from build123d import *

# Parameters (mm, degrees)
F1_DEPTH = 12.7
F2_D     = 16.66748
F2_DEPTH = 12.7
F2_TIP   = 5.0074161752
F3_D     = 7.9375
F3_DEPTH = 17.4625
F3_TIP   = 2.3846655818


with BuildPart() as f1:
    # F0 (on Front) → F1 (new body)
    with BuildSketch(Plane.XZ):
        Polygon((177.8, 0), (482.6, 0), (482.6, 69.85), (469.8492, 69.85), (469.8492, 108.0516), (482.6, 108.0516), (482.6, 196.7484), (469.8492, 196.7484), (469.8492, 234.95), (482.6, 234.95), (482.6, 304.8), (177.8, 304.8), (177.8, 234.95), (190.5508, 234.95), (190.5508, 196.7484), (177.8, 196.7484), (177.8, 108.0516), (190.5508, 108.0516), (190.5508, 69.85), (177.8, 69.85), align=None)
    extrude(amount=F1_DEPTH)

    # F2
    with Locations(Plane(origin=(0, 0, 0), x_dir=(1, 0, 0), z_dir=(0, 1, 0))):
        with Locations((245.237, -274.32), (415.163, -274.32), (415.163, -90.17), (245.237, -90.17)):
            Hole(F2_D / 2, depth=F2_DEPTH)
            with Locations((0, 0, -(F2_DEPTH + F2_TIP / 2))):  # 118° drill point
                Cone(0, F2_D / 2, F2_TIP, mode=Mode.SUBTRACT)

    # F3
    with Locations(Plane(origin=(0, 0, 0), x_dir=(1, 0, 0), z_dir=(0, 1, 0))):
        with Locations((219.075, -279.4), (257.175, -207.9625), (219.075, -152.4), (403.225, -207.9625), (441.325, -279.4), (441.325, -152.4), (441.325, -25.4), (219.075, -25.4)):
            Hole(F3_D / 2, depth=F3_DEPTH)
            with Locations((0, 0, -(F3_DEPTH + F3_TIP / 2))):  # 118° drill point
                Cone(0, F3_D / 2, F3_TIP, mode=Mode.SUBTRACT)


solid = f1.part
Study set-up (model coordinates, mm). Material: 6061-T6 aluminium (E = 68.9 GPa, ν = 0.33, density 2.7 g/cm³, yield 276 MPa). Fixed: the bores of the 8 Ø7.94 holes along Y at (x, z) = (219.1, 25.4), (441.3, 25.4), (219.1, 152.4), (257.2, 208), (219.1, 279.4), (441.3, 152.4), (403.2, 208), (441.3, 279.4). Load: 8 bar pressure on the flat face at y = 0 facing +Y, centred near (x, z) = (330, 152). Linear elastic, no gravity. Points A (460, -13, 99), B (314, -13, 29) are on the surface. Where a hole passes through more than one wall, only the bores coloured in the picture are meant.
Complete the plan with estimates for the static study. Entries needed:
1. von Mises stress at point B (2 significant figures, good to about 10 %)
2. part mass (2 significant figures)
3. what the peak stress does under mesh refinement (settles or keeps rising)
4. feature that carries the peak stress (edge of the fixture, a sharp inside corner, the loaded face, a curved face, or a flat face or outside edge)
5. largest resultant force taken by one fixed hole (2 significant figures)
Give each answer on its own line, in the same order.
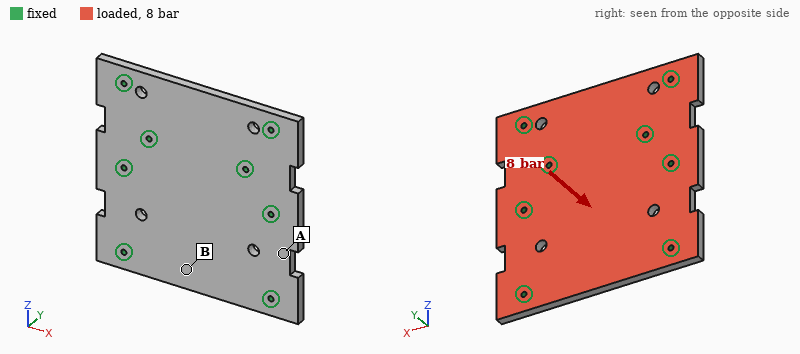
62 MPa
3.1 kg
keeps rising
edge of the fixture
11 kN
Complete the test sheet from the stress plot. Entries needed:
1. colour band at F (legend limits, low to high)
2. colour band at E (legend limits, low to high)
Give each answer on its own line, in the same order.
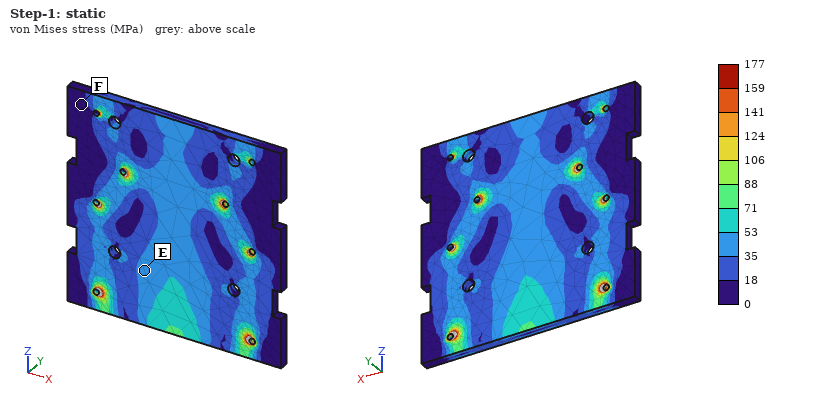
0 to 18 MPa
35 to 53 MPa
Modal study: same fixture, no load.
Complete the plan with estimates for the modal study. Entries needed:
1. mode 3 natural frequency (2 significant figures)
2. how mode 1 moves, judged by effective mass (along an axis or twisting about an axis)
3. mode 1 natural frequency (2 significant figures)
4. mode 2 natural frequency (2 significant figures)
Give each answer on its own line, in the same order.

2000 Hz
along Y
1200 Hz
1600 Hz
